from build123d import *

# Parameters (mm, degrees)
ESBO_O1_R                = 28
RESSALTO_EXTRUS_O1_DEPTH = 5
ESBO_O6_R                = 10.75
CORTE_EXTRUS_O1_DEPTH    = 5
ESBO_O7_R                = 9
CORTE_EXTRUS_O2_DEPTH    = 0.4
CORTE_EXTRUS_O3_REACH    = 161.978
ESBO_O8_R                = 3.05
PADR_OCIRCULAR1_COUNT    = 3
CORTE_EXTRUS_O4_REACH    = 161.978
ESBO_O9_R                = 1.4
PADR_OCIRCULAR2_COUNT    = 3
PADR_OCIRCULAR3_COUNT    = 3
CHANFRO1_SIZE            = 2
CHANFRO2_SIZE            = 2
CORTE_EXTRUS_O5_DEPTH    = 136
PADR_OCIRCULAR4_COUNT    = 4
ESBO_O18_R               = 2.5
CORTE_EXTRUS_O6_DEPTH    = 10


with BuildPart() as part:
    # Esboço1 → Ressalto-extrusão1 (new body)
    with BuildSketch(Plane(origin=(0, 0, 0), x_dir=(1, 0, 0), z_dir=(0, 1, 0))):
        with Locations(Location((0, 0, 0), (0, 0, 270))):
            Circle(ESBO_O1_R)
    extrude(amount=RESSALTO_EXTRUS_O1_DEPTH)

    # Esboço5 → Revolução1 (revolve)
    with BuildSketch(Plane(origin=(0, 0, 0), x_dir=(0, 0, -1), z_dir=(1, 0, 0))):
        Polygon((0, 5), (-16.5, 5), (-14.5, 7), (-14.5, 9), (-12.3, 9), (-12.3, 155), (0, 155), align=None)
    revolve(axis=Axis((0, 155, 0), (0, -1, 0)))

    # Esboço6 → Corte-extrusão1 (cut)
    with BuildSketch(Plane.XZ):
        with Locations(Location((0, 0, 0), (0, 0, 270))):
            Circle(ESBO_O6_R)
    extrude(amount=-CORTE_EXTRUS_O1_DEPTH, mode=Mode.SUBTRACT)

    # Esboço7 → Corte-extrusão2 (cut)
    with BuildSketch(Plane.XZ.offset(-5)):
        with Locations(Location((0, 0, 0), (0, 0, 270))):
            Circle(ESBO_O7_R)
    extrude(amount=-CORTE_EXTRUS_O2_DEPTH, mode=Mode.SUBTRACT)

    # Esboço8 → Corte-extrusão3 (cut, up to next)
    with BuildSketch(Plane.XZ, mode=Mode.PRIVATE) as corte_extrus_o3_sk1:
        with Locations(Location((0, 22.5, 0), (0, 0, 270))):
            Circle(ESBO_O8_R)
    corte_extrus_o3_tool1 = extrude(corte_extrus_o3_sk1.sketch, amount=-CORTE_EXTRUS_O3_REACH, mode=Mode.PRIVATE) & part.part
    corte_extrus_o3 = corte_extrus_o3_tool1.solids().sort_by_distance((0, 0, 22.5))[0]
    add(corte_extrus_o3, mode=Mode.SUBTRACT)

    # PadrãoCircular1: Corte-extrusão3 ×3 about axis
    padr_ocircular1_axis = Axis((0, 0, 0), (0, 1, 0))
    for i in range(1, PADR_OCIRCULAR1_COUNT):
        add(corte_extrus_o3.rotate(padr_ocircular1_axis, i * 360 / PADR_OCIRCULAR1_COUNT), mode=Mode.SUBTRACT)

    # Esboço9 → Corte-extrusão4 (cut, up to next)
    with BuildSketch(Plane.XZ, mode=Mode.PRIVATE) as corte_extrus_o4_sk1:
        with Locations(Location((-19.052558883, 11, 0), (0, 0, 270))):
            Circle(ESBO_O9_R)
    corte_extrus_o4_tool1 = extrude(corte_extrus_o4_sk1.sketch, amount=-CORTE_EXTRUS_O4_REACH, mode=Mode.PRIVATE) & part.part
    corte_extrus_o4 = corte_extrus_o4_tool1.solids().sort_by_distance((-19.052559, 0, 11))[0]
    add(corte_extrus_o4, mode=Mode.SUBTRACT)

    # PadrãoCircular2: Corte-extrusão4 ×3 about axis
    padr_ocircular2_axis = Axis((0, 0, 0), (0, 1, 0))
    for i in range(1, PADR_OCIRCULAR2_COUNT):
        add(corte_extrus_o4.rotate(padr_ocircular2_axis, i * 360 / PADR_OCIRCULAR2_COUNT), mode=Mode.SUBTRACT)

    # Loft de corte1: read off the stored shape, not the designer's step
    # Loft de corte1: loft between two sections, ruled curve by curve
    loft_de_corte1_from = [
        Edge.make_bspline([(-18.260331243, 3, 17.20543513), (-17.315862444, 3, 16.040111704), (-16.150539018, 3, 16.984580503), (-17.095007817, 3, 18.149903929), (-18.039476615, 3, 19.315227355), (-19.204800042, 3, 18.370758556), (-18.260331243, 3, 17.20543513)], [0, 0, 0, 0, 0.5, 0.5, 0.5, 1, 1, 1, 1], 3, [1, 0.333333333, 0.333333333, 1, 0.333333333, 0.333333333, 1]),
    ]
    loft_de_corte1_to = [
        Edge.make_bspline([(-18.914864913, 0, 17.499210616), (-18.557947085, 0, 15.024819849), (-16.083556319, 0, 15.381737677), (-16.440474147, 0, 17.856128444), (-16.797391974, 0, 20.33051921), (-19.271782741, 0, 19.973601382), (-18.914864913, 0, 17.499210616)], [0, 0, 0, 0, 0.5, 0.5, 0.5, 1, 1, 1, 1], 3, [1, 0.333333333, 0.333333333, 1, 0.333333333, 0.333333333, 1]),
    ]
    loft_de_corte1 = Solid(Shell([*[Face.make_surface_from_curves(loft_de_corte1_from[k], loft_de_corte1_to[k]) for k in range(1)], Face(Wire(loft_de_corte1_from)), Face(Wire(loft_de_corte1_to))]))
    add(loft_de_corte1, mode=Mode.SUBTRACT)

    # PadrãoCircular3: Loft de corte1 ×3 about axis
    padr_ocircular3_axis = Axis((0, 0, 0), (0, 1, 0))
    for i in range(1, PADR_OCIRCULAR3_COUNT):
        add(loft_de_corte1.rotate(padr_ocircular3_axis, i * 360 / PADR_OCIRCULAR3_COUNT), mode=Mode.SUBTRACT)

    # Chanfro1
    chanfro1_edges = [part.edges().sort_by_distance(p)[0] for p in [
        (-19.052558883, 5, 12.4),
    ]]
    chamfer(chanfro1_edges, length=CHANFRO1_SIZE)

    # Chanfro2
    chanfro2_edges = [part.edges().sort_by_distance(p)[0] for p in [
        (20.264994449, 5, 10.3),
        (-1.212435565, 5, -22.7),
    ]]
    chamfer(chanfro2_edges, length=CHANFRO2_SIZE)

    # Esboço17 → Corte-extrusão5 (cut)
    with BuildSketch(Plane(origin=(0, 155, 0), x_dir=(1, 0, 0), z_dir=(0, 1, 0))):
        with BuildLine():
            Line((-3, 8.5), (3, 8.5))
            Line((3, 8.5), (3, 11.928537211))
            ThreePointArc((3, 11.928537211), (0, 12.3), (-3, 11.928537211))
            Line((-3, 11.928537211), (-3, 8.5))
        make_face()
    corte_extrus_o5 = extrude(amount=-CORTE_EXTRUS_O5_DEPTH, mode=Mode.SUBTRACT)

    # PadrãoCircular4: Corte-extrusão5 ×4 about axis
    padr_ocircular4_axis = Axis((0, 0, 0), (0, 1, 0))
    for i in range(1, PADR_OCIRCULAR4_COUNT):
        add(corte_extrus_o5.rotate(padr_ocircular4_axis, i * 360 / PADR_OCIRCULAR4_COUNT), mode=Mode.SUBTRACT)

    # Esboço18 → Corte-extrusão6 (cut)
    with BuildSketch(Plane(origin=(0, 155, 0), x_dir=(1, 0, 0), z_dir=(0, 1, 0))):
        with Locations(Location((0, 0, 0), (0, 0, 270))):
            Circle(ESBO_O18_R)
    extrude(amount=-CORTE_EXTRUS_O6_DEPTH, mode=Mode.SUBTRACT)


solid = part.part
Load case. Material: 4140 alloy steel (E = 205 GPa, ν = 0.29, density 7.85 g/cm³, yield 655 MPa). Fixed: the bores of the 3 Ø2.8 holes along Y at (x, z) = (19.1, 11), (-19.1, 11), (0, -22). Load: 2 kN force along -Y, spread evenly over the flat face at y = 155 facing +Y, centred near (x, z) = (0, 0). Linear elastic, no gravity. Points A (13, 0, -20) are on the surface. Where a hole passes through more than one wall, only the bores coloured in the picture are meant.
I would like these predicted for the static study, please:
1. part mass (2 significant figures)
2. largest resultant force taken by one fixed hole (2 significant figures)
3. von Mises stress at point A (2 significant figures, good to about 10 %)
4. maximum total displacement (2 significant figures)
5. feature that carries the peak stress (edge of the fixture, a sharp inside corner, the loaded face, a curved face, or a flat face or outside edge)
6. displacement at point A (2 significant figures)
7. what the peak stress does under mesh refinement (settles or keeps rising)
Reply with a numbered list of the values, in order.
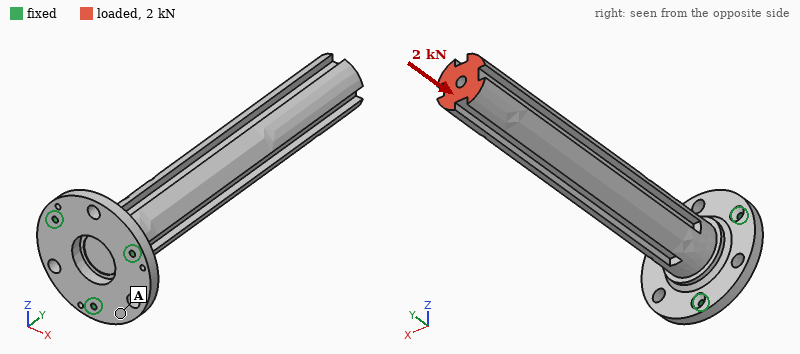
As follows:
1. 550 g
2. 900 N
3. 7.7 MPa
4. 7.5 µm
5. edge of the fixture
6. 2.4 µm
7. keeps rising
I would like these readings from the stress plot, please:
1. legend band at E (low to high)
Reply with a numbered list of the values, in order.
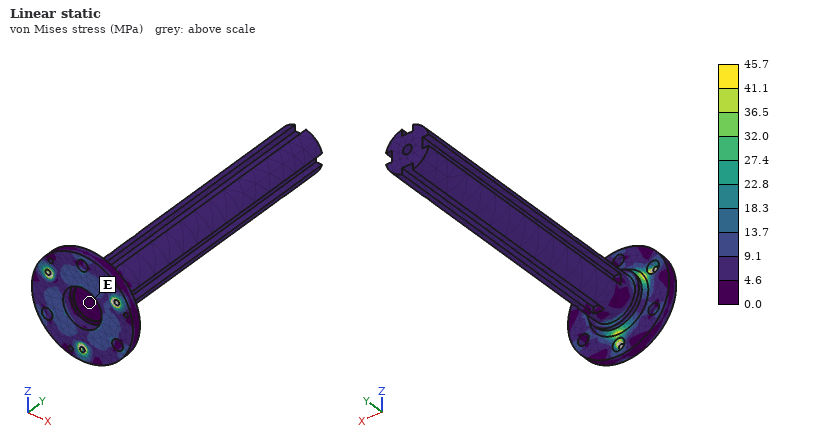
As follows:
1. 0.0 to 4.6 MPa
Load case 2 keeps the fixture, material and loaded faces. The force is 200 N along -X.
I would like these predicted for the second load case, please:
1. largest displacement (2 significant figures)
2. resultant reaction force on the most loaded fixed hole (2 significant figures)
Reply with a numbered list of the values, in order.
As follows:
1. 0.13 mm
2. 1.0 kN
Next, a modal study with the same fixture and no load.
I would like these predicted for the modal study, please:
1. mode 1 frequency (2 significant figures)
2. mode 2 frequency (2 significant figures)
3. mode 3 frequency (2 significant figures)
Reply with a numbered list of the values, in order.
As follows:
1. 560 Hz
2. 560 Hz
3. 3600 Hz
